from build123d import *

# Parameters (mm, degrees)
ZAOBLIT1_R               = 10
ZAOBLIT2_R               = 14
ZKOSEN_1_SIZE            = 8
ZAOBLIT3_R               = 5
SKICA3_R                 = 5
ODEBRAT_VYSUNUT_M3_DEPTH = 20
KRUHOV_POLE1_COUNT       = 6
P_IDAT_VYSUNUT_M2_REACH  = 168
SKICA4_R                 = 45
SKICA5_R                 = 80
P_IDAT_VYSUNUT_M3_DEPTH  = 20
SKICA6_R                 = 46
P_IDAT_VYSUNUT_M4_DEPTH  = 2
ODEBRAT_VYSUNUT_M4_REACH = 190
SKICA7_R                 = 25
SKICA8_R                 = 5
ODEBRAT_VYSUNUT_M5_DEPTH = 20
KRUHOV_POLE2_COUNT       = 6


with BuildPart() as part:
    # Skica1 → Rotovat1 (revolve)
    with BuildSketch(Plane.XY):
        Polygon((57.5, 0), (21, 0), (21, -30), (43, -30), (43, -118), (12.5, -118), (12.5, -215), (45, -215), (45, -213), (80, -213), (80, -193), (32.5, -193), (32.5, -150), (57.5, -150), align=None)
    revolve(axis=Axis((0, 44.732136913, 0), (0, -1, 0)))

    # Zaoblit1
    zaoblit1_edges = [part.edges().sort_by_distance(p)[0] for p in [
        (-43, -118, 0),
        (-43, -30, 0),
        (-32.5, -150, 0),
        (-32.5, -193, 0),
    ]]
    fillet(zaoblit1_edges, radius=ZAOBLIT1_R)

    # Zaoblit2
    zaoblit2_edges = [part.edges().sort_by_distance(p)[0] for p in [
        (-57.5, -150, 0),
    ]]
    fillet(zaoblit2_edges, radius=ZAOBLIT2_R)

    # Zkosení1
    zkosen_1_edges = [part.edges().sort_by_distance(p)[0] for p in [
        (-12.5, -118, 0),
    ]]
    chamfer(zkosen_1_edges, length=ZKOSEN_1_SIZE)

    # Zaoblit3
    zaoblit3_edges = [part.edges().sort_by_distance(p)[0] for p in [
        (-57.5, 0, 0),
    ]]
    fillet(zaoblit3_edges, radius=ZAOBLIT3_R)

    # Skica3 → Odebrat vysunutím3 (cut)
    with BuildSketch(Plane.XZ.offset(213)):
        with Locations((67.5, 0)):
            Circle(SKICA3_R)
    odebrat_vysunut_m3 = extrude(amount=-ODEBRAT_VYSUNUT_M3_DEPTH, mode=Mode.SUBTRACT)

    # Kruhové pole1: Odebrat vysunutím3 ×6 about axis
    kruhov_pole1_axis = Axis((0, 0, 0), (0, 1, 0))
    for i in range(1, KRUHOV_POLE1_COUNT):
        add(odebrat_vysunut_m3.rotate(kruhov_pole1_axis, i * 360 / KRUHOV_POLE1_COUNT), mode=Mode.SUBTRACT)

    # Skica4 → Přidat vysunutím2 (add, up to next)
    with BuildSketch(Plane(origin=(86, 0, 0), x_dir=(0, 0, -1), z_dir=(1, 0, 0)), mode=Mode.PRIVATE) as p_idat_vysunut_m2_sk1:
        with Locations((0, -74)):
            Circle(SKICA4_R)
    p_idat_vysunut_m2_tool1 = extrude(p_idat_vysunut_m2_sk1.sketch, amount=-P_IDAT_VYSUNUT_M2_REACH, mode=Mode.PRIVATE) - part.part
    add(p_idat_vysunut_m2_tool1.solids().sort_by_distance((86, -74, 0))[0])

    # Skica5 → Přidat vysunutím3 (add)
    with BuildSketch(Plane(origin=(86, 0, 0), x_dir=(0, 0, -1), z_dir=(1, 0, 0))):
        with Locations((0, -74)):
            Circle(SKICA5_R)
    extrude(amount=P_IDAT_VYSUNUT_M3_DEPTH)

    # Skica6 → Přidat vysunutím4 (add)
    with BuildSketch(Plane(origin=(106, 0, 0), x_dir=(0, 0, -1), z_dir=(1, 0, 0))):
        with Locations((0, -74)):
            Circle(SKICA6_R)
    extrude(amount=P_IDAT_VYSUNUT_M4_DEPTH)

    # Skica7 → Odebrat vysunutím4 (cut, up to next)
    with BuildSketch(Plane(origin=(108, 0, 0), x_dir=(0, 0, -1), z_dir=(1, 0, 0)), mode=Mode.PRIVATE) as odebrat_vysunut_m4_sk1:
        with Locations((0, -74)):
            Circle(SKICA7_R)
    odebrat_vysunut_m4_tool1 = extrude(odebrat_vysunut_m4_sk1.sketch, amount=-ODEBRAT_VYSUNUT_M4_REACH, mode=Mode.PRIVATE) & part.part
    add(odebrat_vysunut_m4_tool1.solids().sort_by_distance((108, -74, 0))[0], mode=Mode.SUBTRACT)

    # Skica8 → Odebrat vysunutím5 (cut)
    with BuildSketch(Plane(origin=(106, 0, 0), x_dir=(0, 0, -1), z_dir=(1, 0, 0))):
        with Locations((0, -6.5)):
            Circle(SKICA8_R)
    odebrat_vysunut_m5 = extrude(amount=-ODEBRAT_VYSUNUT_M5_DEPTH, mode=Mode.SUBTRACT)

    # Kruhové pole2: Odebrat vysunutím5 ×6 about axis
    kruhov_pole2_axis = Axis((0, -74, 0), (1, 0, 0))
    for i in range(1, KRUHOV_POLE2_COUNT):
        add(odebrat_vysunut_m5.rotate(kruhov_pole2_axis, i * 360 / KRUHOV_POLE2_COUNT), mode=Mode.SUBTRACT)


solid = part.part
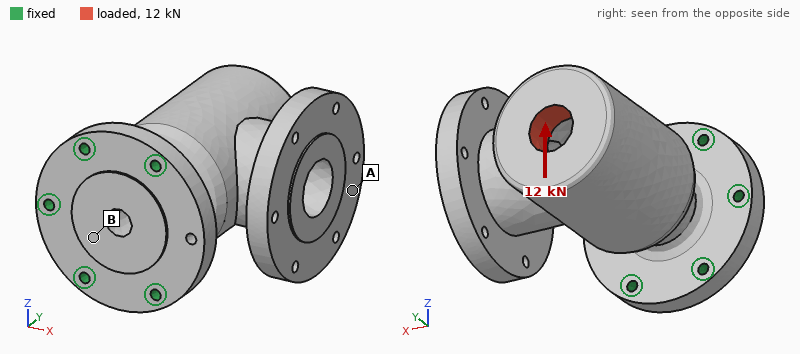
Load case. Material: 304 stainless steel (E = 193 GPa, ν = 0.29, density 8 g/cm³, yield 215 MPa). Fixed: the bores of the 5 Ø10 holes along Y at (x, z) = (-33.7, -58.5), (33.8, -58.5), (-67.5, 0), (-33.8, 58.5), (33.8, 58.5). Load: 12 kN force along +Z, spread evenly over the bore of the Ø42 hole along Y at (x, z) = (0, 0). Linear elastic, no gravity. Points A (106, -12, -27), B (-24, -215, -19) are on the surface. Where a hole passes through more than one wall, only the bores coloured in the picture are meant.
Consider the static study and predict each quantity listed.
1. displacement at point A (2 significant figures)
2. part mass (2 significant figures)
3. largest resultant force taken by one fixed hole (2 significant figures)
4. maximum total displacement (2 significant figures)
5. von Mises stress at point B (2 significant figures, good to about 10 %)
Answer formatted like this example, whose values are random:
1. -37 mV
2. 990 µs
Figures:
1. 0.19 mm
2. 16 kg
3. 12 kN
4. 0.21 mm
5. 30 MPa
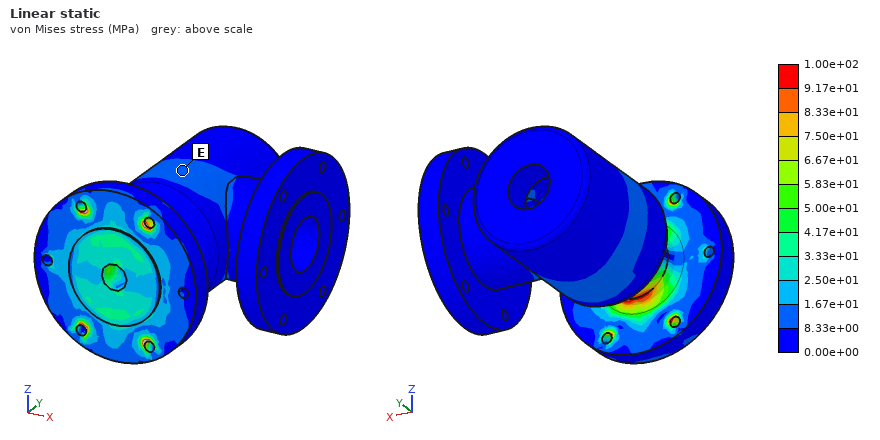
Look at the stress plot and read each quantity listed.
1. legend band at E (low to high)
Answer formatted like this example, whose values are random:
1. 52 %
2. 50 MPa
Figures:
1. 8.33e+00 to 1.67e+01 MPa
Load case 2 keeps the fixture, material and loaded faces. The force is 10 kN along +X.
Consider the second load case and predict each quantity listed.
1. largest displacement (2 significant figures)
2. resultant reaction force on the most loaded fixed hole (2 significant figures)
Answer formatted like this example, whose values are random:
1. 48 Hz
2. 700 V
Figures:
1. 0.23 mm
2. 12 kN
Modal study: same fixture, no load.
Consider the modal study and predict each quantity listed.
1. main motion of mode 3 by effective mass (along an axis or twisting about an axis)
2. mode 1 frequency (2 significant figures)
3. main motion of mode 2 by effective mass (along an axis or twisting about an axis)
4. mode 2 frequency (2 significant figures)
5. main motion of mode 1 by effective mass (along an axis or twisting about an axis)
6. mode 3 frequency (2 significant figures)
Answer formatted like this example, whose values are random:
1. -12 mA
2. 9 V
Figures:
1. twisting about Y
2. 440 Hz
3. along Z
4. 500 Hz
5. along X
6. 1100 Hz
